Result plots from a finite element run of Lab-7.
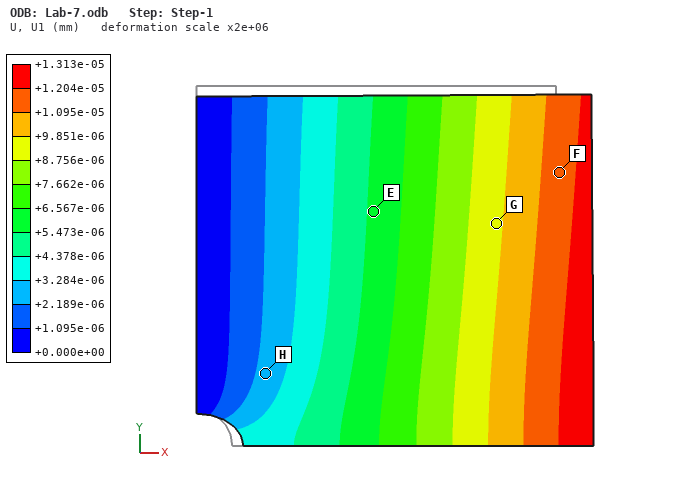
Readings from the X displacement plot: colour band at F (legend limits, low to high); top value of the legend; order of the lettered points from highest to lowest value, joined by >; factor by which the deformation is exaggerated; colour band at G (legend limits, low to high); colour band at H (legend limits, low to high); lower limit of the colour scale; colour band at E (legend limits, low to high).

+1.095e-05 to +1.204e-05 mm
+1.313e-05 mm
F > G > E > H
2e+06
+8.756e-06 to +9.851e-06 mm
+2.189e-06 to +3.284e-06 mm
+0.000e+00 mm
+5.473e-06 to +6.567e-06 mm
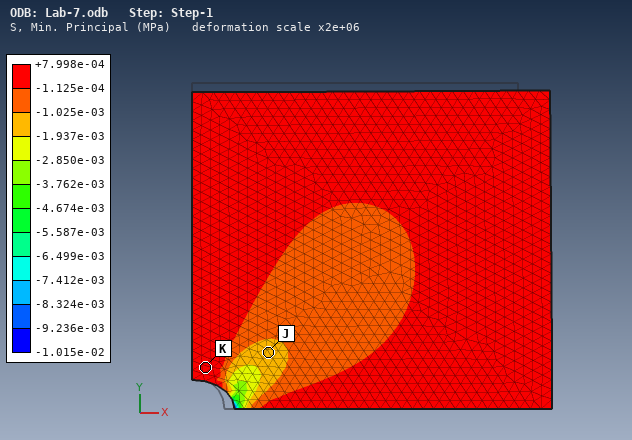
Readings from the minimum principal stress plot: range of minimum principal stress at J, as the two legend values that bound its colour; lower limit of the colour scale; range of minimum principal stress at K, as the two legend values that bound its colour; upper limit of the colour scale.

-1.937e-03 to -1.025e-03 MPa
-1.015e-02 MPa
-1.125e-04 to +7.998e-04 MPa
+7.998e-04 MPa
